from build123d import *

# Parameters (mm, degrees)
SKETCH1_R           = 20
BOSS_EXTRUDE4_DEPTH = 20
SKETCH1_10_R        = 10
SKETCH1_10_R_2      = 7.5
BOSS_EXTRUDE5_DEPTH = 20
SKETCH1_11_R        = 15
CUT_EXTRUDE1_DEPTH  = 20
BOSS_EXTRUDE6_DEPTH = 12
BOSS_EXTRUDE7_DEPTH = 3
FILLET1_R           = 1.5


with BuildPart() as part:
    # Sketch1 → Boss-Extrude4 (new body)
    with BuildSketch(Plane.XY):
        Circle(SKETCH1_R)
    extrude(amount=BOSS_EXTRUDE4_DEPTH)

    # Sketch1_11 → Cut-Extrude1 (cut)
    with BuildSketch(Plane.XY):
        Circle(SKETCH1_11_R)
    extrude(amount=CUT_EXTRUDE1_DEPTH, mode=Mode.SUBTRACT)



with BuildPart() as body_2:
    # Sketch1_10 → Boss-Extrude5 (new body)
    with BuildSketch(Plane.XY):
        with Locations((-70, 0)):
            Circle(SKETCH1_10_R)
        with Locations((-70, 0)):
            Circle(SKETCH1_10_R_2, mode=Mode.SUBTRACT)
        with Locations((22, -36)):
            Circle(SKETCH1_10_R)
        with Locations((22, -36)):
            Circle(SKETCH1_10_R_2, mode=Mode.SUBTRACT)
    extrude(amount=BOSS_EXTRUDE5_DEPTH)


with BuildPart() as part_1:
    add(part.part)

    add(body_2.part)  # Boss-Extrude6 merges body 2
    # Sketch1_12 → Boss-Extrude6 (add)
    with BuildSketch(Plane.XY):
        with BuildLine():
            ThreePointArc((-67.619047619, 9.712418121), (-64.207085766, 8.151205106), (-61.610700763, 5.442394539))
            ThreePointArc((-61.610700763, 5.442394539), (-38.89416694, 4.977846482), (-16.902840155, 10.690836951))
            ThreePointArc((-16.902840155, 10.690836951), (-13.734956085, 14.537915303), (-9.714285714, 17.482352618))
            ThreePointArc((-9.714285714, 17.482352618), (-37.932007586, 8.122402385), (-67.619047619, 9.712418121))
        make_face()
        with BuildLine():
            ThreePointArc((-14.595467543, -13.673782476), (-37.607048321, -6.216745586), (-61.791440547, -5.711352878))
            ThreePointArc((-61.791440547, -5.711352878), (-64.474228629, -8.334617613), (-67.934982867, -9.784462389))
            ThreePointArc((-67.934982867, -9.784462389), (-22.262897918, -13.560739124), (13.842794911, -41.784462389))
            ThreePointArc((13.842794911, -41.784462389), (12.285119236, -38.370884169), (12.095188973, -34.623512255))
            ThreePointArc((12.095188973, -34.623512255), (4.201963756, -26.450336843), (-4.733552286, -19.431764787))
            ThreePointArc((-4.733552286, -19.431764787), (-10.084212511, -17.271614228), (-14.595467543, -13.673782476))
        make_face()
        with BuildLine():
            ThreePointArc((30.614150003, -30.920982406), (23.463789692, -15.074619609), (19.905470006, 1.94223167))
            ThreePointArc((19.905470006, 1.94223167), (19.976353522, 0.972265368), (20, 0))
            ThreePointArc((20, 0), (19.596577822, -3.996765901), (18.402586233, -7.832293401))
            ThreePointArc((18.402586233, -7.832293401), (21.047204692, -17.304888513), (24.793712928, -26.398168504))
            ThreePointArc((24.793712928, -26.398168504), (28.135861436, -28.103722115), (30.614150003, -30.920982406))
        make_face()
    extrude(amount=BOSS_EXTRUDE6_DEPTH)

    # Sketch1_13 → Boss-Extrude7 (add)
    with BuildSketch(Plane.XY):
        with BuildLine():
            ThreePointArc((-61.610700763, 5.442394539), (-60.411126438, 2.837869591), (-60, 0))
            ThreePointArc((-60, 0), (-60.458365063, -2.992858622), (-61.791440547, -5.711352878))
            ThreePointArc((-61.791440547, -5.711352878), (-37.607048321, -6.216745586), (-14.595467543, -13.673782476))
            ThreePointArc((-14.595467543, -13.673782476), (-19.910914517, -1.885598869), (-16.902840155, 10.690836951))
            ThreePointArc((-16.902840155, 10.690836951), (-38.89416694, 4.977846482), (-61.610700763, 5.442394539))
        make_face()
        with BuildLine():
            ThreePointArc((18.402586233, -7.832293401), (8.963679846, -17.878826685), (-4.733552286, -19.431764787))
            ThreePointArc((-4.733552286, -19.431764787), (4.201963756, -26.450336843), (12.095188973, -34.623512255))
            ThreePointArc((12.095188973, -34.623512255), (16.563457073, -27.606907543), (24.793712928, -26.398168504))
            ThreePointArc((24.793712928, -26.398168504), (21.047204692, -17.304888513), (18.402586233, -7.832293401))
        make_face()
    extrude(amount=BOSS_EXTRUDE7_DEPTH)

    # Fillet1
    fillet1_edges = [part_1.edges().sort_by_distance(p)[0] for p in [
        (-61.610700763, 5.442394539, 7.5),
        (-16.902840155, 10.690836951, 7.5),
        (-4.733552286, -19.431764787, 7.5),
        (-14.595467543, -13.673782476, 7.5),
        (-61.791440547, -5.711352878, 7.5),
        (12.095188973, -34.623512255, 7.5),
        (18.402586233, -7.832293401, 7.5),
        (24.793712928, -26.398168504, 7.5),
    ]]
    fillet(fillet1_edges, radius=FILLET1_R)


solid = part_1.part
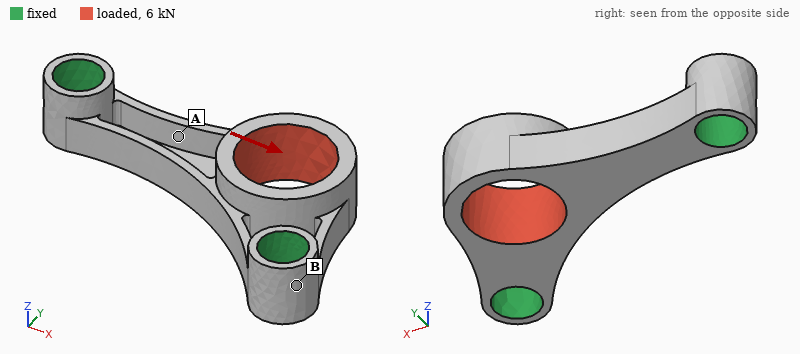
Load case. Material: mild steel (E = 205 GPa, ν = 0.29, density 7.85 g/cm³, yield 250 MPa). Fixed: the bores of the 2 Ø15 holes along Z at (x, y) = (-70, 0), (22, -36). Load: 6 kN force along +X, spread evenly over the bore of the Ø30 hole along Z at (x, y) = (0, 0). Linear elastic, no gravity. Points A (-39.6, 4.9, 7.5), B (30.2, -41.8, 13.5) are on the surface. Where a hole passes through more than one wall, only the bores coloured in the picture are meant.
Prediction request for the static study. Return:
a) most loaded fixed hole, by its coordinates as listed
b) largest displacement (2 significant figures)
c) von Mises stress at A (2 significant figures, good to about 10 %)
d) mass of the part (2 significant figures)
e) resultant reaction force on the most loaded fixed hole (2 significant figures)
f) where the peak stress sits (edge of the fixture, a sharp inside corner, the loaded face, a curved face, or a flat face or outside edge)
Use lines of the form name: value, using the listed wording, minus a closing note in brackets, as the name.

most loaded fixed hole, by its coordinates as listed: (-70, 0)
largest displacement: 64 µm
von Mises stress at A: 55 MPa
mass of the part: 190 g
resultant reaction force on the most loaded fixed hole: 4.4 kN
where the peak stress sits: a curved face
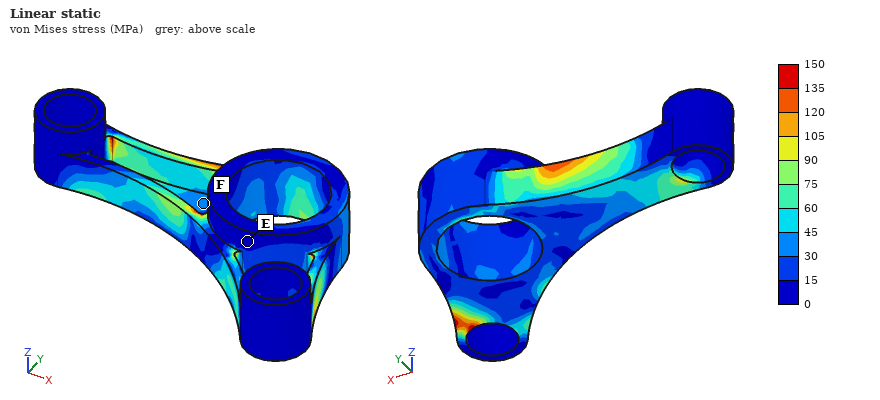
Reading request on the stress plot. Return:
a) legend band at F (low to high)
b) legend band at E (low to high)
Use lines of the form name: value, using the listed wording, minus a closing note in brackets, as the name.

legend band at F: 30 to 45 MPa
legend band at E: 0 to 15 MPa
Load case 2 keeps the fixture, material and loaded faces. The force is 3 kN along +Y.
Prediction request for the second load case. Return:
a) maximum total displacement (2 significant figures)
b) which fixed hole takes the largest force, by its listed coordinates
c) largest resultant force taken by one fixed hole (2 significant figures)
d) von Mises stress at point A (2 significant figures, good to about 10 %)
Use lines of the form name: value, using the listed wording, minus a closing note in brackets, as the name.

maximum total displacement: 64 µm
which fixed hole takes the largest force, by its listed coordinates: (22, -36)
largest resultant force taken by one fixed hole: 3.1 kN
von Mises stress at point A: 19 MPa
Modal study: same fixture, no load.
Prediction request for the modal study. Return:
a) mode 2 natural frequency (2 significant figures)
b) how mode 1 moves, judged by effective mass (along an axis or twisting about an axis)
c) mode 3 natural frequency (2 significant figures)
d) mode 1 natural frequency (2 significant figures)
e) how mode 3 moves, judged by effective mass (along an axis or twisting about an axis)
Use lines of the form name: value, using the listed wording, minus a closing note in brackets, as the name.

mode 2 natural frequency: 5700 Hz
how mode 1 moves, judged by effective mass: along Z
mode 3 natural frequency: 8200 Hz
mode 1 natural frequency: 2500 Hz
how mode 3 moves, judged by effective mass: along Y
